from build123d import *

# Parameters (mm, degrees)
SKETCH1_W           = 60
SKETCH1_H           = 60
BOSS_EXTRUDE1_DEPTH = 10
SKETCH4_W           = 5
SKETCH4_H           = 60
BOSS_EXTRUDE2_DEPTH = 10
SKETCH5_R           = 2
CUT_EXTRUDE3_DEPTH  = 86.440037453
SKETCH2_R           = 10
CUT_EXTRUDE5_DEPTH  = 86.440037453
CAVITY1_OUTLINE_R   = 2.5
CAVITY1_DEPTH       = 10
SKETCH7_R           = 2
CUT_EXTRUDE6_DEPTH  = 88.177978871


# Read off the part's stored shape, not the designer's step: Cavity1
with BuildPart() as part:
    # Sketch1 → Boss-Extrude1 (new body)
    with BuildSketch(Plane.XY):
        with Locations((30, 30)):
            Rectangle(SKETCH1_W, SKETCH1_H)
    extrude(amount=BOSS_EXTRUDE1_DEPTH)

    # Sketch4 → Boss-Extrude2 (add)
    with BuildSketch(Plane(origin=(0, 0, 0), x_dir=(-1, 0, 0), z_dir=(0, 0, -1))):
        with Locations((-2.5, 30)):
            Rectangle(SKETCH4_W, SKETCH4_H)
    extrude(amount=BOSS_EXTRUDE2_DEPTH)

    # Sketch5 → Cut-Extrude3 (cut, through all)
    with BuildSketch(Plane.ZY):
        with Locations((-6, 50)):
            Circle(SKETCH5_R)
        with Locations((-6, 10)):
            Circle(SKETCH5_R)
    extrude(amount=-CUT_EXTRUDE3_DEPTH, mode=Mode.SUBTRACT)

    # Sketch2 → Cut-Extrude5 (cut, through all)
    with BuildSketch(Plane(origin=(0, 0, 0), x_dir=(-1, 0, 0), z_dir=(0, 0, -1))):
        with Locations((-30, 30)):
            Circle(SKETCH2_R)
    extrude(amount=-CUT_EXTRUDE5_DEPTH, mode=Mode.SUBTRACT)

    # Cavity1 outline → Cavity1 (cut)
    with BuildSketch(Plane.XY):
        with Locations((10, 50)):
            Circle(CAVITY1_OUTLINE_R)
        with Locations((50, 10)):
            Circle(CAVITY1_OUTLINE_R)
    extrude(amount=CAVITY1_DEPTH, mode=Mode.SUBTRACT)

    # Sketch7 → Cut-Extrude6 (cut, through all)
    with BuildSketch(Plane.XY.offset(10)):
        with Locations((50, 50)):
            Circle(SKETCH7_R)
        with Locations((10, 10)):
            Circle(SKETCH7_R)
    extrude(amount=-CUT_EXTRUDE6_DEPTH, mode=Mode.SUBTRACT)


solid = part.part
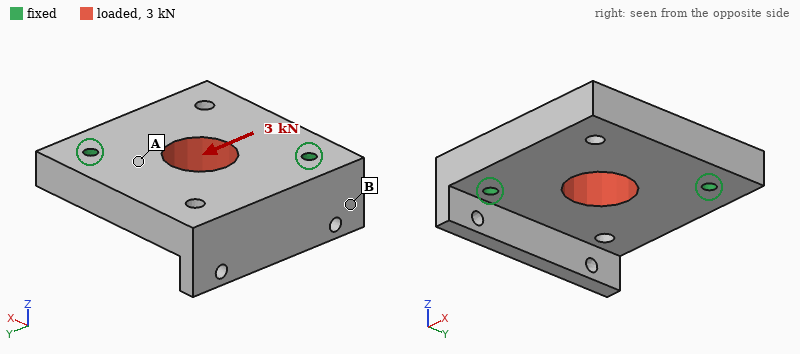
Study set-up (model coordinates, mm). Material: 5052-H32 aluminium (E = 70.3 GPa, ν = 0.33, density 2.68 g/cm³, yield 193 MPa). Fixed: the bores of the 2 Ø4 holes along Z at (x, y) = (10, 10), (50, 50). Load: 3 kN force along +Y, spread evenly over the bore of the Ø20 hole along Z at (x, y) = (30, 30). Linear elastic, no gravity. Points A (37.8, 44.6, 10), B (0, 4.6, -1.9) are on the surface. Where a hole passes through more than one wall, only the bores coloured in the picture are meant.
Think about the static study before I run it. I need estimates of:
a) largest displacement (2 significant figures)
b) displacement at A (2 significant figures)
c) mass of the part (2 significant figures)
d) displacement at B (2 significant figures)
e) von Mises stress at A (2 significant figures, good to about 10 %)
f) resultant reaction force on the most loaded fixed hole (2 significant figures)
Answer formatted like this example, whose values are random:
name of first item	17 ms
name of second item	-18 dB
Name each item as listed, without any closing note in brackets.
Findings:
largest displacement	4.0 µm
displacement at A	2.7 µm
mass of the part	94 g
displacement at B	0.61 µm
von Mises stress at A	5.2 MPa
resultant reaction force on the most loaded fixed hole	1.5 kN
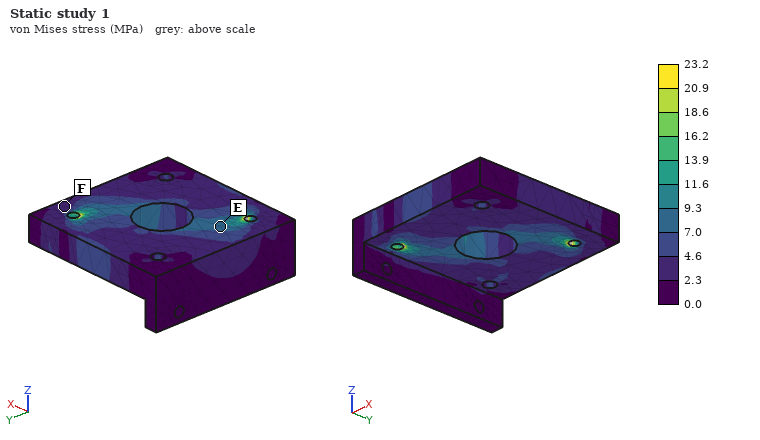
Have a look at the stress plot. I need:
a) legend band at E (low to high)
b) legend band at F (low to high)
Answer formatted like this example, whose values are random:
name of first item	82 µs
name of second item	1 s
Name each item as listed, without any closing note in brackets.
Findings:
legend band at E	7.0 to 9.3 MPa
legend band at F	2.3 to 4.6 MPa
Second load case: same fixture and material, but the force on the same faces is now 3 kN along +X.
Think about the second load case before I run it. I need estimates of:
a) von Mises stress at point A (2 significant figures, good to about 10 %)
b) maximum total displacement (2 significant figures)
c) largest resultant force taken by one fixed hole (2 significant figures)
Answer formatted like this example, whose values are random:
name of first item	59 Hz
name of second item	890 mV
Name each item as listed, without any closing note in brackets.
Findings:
von Mises stress at point A	7.4 MPa
maximum total displacement	3.9 µm
largest resultant force taken by one fixed hole	1.5 kN
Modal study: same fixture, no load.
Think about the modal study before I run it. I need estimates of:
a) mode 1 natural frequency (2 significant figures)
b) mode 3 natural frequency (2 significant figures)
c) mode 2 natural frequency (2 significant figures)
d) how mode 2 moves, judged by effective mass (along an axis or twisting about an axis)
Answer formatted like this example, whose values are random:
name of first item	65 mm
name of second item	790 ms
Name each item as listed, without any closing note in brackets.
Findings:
mode 1 natural frequency	4500 Hz
mode 3 natural frequency	13 kHz
mode 2 natural frequency	5800 Hz
how mode 2 moves, judged by effective mass	along Z
